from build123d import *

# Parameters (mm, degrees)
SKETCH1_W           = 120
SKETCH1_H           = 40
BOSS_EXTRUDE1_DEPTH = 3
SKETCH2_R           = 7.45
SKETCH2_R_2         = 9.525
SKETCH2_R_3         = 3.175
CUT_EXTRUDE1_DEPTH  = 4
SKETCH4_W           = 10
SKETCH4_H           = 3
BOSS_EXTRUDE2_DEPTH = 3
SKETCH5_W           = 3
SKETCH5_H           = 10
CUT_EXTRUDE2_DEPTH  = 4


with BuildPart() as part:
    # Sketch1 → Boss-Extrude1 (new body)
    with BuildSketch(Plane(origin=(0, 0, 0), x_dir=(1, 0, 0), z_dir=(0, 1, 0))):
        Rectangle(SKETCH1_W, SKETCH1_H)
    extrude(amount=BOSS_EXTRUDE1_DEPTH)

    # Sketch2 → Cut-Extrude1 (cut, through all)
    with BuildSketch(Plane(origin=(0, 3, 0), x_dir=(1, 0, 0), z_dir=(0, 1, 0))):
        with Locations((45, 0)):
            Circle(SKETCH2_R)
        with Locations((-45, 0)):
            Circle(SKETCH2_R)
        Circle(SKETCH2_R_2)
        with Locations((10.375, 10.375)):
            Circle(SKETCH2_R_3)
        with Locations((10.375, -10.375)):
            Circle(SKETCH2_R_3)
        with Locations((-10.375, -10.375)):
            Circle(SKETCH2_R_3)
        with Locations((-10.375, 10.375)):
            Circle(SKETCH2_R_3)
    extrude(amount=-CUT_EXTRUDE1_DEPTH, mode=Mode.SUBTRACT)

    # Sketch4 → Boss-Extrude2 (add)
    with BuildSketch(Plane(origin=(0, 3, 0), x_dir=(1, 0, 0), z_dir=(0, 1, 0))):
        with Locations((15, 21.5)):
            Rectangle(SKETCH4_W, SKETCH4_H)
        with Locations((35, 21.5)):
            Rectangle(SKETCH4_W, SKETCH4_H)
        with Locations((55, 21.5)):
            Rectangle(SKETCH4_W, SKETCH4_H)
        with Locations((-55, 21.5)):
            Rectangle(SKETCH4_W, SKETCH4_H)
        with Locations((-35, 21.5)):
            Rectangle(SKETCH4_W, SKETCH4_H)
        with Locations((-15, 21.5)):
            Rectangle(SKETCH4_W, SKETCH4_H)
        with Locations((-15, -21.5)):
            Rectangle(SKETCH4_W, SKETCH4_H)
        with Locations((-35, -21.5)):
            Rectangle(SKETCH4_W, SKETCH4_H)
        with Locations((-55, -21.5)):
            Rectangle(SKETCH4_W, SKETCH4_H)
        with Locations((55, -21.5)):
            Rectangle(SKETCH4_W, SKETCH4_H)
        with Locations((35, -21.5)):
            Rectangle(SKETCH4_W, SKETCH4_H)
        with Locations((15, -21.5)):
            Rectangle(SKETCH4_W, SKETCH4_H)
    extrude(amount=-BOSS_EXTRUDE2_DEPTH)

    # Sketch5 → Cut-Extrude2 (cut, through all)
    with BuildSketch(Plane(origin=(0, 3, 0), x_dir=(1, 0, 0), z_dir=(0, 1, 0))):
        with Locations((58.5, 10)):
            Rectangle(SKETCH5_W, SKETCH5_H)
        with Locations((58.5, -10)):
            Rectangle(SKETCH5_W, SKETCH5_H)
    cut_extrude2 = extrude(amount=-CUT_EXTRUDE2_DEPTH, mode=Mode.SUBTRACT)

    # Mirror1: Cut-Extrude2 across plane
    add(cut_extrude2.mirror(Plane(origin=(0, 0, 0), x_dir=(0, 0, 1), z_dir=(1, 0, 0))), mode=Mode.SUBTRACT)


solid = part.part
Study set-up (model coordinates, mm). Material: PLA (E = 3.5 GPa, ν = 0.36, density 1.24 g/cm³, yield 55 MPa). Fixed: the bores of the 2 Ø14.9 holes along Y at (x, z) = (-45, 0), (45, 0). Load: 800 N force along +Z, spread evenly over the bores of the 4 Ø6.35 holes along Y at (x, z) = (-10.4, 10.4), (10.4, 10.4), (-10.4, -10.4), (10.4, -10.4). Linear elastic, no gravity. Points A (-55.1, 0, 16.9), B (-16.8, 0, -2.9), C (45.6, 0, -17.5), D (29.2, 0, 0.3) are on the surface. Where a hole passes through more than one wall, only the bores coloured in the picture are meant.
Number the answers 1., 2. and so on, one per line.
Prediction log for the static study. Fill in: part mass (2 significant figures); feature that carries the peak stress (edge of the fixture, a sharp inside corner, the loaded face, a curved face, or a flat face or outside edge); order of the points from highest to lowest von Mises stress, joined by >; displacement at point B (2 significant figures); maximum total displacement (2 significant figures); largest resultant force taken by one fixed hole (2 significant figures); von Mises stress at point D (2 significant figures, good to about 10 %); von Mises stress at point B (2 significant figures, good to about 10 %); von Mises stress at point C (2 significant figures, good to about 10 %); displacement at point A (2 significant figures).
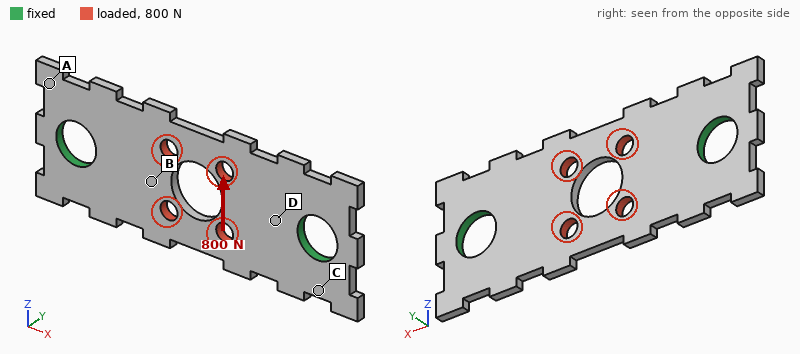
1. 16 g
2. edge of the fixture
3. D > B > C > A
4. 0.13 mm
5. 0.19 mm
6. 400 N
7. 8.4 MPa
8. 6.6 MPa
9. 3.3 MPa
10. 0.033 mm
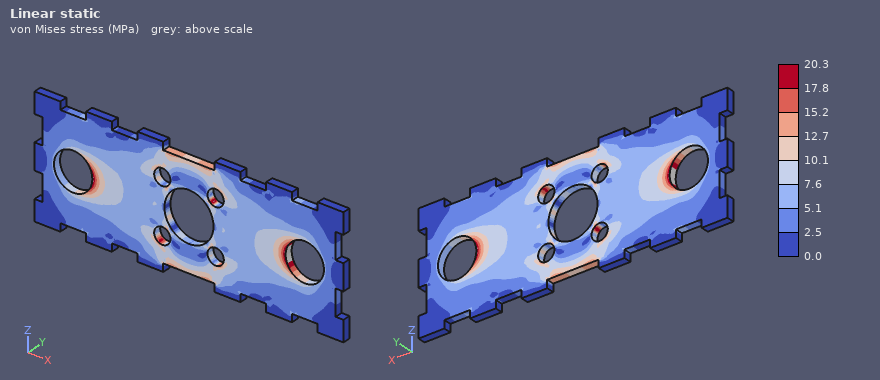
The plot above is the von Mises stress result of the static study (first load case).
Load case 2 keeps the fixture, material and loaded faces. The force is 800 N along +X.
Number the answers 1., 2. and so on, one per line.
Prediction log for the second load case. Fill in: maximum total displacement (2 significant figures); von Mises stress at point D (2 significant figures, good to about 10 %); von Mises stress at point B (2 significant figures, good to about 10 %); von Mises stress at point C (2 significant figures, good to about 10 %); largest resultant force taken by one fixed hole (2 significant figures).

1. 55 µm
2. 4.7 MPa
3. 3.5 MPa
4. 1.1 MPa
5. 400 N
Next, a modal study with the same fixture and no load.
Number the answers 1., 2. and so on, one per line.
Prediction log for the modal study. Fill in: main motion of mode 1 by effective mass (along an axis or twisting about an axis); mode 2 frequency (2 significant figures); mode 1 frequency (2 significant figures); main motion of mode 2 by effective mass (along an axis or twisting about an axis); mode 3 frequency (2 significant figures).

1. along Y
2. 1000 Hz
3. 820 Hz
4. twisting about X
5. 1900 Hz
